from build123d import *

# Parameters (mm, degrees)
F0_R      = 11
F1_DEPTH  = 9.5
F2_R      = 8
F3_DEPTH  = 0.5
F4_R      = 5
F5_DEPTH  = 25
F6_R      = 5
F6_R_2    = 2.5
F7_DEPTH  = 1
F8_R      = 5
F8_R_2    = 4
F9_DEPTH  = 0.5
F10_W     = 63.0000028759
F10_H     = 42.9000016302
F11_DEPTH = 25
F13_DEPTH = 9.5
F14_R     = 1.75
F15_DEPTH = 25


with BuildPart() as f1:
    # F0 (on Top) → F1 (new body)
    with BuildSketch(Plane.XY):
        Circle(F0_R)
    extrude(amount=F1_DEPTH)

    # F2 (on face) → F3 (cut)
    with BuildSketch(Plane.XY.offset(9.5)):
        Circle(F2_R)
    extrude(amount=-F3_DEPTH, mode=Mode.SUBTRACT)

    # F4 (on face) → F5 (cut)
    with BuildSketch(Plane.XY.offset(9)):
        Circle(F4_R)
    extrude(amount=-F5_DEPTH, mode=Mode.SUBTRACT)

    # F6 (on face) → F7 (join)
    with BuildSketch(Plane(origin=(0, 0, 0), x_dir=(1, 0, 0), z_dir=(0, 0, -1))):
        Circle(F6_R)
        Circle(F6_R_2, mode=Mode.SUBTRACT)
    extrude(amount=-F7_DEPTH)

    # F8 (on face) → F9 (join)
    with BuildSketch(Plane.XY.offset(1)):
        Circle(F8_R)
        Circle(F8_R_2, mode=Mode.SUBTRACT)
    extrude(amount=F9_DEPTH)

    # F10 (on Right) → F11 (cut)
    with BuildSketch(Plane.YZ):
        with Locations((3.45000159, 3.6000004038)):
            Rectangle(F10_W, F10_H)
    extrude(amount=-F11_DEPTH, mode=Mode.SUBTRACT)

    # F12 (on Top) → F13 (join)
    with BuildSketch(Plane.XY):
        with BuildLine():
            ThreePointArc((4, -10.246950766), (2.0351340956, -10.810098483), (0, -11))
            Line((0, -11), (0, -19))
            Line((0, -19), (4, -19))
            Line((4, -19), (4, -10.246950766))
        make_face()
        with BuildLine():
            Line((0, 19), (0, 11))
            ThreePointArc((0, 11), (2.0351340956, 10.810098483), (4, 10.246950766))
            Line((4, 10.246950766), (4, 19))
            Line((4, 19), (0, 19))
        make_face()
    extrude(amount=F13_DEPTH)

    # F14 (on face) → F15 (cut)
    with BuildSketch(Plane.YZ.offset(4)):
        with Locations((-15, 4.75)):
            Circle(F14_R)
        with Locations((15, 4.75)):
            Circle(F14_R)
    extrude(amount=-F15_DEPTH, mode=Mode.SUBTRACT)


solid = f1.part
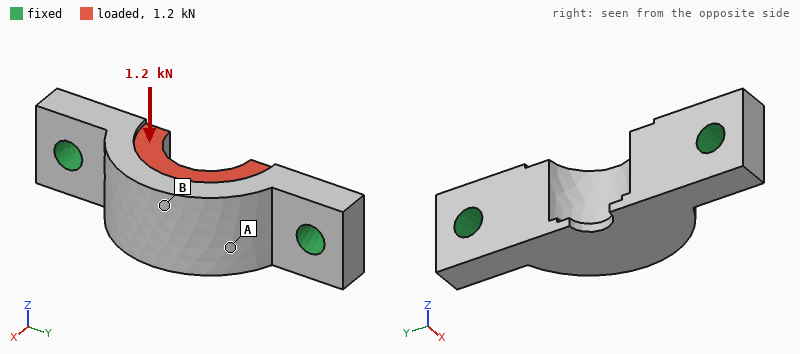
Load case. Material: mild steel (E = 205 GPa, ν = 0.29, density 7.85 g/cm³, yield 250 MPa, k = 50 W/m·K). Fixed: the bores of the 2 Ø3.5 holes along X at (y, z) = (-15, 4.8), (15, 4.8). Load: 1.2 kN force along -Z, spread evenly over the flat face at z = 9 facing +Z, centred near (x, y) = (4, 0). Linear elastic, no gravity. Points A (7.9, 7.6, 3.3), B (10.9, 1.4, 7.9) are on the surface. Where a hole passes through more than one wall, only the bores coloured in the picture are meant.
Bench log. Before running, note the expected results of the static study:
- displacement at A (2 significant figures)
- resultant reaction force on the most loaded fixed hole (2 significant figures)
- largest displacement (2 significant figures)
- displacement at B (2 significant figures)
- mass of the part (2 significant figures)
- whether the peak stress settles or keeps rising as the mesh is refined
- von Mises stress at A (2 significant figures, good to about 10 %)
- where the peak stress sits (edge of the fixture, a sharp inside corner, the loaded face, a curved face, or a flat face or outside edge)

6.7 µm
600 N
10 µm
9.9 µm
16 g
keeps rising
32 MPa
edge of the fixture
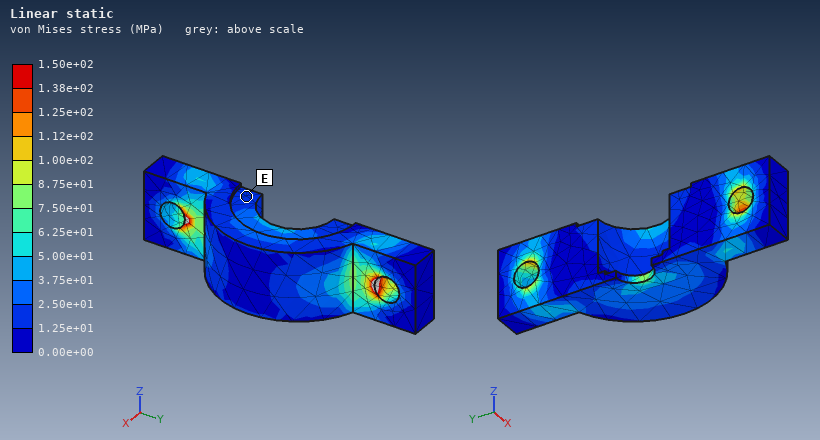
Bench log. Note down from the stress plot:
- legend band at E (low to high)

1.25e+01 to 2.50e+01 MPa
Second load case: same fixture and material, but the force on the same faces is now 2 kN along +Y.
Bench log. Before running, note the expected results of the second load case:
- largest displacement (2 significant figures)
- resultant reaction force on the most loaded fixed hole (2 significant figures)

3.3 µm
1.1 kN
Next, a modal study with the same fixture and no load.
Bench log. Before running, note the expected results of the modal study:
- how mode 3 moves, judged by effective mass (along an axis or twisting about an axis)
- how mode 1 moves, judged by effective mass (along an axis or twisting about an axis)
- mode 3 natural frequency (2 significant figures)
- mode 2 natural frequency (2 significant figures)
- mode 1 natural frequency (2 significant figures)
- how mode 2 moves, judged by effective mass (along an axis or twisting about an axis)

along Z
along Z
43 kHz
29 kHz
17 kHz
along X
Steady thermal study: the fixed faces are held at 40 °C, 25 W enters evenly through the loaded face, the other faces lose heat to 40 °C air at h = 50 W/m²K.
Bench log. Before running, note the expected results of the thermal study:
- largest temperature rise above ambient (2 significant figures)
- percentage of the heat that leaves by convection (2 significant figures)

71 K
7.6 %
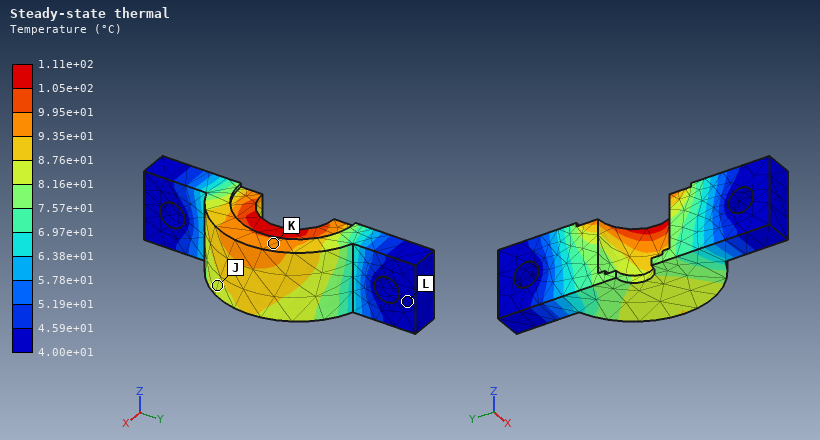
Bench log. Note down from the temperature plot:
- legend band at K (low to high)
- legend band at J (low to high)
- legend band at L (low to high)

9.35e+01 to 9.95e+01 °C
8.16e+01 to 8.76e+01 °C
4.00e+01 to 4.59e+01 °C
